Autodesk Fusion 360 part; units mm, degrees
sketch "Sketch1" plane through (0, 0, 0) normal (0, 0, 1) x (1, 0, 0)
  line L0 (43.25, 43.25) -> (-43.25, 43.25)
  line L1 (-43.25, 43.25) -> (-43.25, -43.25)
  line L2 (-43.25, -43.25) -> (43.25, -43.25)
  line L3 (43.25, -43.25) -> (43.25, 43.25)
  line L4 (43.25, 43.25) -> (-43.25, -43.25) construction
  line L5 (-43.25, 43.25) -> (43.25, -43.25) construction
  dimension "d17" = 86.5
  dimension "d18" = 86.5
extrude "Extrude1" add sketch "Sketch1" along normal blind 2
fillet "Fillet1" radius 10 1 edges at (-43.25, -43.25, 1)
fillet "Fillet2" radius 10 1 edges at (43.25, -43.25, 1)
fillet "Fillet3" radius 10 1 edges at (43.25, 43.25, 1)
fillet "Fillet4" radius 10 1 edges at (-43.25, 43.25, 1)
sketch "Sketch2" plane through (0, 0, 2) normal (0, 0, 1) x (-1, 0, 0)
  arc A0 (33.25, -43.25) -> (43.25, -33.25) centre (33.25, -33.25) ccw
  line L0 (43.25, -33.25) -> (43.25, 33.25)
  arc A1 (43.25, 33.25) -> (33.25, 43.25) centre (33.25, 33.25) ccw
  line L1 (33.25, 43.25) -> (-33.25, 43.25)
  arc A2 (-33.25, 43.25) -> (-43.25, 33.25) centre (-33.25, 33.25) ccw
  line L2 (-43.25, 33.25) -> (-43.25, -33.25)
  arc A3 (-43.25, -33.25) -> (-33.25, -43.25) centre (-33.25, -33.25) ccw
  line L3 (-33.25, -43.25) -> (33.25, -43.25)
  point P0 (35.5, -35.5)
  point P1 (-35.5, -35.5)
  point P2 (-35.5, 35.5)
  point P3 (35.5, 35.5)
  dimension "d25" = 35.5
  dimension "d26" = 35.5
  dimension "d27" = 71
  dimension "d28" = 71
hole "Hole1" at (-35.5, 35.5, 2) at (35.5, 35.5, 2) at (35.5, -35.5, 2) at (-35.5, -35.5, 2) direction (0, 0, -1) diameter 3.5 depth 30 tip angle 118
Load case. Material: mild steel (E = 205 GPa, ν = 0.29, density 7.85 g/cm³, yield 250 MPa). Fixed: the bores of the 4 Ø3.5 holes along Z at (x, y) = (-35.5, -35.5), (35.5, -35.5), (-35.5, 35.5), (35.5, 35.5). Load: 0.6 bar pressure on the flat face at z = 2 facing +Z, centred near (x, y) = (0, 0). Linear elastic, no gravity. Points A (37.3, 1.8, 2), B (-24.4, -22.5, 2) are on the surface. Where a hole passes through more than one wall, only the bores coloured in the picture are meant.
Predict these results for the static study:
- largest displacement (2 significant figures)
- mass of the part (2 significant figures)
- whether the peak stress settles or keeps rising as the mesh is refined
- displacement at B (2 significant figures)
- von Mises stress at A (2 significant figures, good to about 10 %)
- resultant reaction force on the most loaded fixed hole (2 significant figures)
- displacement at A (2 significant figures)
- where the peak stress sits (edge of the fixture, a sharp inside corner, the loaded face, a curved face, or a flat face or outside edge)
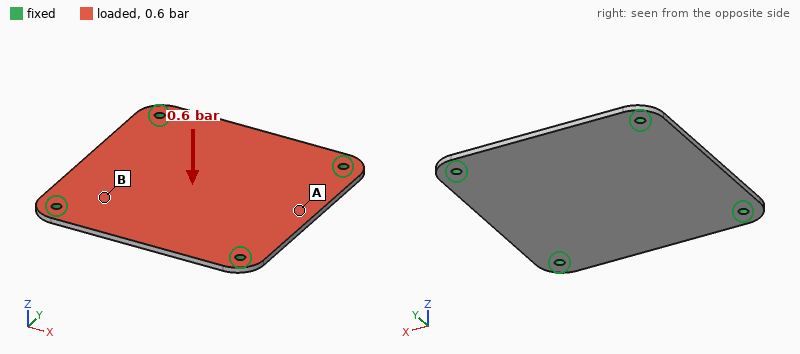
77 µm
120 g
keeps rising
32 µm
25 MPa
110 N
39 µm
edge of the fixture
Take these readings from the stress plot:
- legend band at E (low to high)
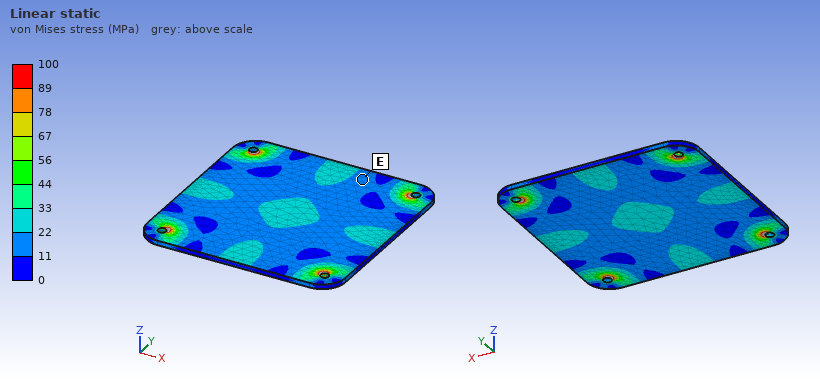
11 to 22 MPa
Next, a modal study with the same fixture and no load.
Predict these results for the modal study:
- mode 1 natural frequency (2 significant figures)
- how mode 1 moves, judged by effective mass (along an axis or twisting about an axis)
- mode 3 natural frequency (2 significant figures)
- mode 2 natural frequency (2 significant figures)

1400 Hz
along Z
2300 Hz
2300 Hz
